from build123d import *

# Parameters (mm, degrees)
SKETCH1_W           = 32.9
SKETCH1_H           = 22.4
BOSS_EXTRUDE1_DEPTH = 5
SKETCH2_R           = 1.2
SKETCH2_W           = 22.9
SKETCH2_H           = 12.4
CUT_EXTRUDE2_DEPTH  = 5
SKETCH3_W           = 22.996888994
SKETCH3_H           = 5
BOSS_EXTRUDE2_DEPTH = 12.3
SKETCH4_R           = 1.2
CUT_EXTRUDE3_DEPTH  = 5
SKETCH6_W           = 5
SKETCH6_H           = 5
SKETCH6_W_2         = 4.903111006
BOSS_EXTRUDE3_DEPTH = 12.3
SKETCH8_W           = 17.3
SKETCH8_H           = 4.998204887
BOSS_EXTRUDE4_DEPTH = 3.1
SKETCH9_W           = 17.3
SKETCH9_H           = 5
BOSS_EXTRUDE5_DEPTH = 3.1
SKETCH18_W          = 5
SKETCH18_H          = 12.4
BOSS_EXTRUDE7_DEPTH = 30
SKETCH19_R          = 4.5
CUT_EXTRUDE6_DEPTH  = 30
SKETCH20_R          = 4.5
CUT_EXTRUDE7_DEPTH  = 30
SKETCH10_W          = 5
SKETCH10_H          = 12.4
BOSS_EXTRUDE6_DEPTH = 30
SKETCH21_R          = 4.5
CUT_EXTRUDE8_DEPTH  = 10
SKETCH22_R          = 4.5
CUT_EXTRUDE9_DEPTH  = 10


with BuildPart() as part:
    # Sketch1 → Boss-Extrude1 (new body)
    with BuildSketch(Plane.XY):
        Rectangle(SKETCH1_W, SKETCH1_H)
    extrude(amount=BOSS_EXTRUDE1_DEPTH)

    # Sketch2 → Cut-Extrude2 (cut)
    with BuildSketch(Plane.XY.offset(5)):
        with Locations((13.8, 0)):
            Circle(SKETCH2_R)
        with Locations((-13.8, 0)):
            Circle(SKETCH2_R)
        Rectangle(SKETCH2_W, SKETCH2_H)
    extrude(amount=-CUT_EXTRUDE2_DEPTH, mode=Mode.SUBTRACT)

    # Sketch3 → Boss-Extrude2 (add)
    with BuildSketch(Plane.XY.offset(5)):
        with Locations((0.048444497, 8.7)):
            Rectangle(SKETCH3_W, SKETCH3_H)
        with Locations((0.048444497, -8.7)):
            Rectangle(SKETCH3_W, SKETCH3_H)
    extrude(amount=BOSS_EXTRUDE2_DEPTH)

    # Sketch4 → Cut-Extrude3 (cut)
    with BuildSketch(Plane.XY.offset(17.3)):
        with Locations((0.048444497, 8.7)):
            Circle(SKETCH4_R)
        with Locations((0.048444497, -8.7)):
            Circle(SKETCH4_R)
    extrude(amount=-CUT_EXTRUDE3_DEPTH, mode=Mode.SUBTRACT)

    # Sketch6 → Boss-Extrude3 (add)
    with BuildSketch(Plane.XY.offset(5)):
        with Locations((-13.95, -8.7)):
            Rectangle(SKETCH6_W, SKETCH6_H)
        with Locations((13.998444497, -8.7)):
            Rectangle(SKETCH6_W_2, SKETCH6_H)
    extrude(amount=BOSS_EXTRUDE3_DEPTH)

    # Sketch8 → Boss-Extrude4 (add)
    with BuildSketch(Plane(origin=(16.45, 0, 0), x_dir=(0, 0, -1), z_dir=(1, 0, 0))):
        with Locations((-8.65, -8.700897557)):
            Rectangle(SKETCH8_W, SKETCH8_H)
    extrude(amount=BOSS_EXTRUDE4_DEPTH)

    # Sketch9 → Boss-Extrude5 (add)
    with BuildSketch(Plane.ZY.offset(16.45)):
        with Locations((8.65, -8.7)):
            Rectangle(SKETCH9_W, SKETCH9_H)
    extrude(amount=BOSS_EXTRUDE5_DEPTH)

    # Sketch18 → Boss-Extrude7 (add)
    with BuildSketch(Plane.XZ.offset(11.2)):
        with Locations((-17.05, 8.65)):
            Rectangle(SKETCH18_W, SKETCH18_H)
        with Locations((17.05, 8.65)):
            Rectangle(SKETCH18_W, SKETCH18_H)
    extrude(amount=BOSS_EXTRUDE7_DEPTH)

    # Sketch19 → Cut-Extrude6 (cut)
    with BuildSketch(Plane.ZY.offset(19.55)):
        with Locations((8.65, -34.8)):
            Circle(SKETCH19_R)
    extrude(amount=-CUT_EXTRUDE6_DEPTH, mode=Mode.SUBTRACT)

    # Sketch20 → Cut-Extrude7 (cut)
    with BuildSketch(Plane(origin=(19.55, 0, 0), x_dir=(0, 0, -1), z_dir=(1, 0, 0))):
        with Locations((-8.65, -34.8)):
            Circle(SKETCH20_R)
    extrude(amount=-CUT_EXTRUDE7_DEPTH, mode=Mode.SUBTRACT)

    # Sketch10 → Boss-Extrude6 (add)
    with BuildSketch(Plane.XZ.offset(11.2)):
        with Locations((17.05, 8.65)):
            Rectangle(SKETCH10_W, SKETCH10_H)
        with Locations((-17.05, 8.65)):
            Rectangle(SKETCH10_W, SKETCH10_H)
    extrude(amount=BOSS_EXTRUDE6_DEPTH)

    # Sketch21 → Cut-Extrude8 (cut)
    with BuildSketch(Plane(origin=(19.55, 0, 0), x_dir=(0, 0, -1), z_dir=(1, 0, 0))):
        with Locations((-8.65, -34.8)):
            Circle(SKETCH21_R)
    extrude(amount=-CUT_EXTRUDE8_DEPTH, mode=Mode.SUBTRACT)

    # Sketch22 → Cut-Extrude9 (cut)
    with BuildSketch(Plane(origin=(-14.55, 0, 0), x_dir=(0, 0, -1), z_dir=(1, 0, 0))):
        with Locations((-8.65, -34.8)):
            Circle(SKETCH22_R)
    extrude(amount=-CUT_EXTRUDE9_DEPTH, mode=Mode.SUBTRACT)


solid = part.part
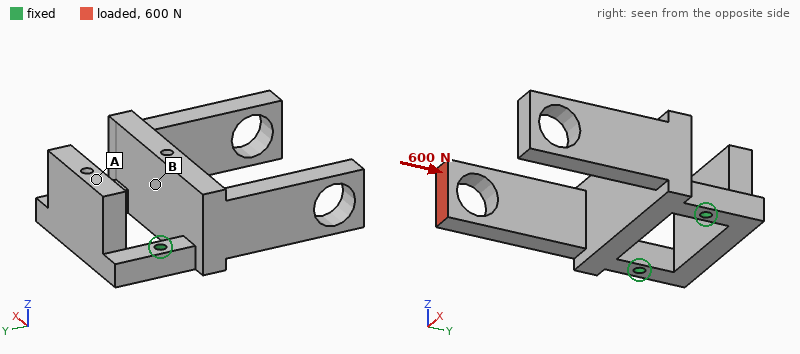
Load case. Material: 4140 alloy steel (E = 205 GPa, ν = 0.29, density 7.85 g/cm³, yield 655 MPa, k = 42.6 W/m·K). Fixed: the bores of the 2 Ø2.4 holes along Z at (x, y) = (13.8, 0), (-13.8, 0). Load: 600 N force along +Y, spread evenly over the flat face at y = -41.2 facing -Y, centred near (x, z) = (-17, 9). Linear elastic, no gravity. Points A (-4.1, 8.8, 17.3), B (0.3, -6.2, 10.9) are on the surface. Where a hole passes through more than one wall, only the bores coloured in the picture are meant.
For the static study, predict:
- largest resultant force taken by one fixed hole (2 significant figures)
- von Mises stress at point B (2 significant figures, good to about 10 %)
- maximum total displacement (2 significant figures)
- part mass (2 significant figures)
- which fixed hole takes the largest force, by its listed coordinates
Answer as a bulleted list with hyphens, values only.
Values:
- 660 N
- 23 MPa
- 71 µm
- 72 g
- (-13.8, 0)
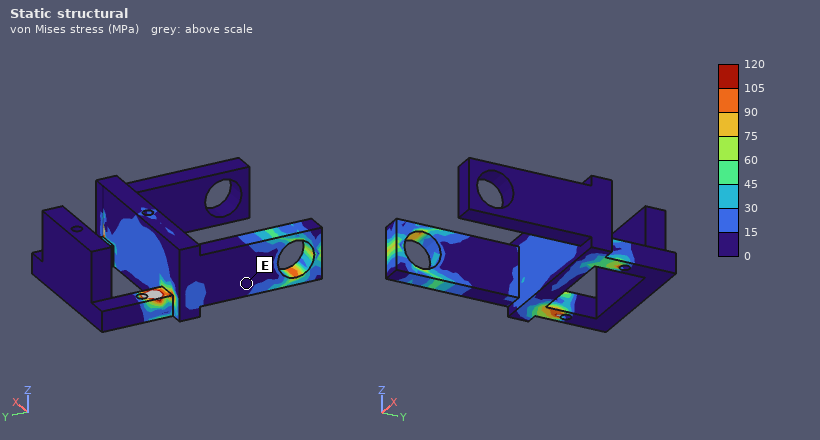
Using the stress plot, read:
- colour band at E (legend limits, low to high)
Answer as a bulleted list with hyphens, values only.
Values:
- 0 to 15 MPa
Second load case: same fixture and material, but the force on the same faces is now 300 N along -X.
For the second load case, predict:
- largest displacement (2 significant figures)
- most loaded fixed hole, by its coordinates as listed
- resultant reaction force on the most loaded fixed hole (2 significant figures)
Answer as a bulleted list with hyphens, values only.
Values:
- 0.20 mm
- (13.8, 0)
- 650 N
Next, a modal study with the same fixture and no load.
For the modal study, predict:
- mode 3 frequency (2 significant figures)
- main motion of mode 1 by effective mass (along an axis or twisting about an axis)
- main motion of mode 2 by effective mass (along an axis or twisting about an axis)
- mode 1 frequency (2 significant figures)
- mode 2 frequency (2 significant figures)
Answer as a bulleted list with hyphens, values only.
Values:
- 3700 Hz
- along Z
- along X
- 2100 Hz
- 3300 Hz
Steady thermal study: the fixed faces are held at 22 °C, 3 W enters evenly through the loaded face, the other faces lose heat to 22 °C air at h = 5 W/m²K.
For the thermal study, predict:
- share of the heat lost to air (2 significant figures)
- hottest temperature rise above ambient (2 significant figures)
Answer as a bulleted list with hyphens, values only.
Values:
- 11 %
- 71 K
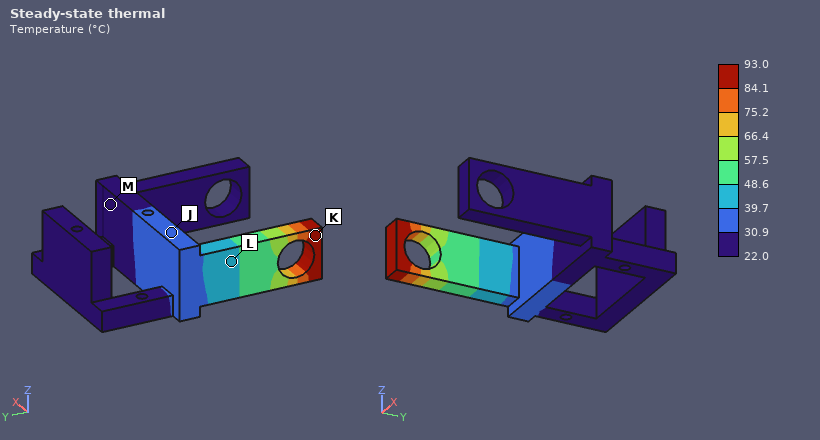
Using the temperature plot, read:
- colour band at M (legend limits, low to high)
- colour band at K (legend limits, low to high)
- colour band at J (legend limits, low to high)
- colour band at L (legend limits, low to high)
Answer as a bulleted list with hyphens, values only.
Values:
- 22.0 to 30.9 °C
- 84.1 to 93.0 °C
- 30.9 to 39.7 °C
- 39.7 to 48.6 °C
